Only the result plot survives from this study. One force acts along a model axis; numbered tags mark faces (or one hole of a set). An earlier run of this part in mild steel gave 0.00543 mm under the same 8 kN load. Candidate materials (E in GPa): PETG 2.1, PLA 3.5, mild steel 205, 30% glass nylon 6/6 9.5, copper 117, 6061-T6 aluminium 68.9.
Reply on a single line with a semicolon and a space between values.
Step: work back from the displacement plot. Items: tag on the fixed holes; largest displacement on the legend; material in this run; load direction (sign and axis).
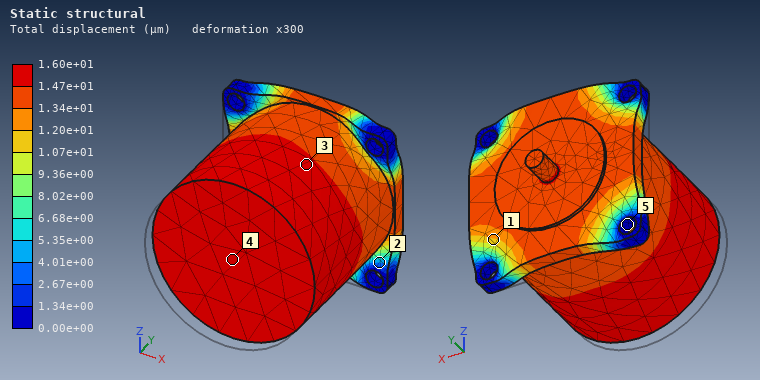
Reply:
5; 1.60e+01 µm; 6061-T6 aluminium; +Y
